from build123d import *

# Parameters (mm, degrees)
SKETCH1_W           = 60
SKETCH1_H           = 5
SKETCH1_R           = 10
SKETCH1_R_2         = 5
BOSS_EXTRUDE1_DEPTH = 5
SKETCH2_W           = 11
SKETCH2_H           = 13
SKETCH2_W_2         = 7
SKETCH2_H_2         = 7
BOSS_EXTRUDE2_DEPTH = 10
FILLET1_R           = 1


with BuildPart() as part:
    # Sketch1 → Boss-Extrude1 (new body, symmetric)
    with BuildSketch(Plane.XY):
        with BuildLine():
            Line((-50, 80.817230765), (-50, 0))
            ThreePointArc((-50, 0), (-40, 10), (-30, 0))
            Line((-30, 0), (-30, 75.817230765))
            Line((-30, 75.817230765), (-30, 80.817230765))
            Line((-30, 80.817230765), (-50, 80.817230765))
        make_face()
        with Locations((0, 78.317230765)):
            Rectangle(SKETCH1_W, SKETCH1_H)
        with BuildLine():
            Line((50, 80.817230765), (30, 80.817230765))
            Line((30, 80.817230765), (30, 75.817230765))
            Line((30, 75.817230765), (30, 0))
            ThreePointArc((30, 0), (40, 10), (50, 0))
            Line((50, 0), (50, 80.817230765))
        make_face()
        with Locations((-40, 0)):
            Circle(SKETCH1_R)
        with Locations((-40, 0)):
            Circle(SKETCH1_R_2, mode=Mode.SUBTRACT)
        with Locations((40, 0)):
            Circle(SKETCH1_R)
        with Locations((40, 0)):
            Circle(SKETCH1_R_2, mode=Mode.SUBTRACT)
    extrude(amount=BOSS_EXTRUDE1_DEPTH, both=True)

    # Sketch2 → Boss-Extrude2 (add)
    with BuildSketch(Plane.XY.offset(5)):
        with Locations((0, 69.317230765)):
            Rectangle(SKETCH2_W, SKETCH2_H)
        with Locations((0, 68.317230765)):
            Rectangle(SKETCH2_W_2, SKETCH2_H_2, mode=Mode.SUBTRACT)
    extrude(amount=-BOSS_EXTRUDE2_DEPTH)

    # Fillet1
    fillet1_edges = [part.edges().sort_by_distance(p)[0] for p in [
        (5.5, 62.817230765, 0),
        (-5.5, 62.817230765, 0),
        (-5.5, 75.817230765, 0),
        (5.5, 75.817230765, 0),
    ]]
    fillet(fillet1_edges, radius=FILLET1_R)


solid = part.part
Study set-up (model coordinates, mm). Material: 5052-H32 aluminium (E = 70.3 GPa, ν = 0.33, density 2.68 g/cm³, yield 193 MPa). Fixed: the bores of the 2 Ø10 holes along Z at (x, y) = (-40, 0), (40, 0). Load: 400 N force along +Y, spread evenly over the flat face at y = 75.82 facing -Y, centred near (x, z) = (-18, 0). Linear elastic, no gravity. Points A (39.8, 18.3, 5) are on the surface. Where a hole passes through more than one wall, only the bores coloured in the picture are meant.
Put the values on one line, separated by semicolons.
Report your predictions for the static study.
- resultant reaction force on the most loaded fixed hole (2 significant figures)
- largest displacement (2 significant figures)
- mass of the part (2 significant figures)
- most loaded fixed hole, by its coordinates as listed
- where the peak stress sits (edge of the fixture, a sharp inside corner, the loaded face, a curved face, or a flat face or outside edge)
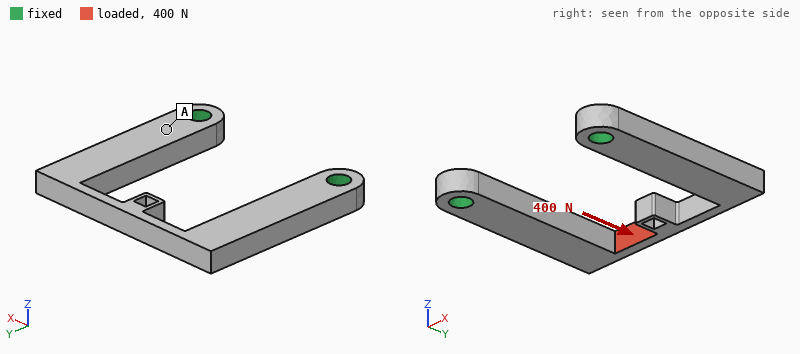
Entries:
340 N; 46 µm; 100 g; (-40, 0); the loaded face
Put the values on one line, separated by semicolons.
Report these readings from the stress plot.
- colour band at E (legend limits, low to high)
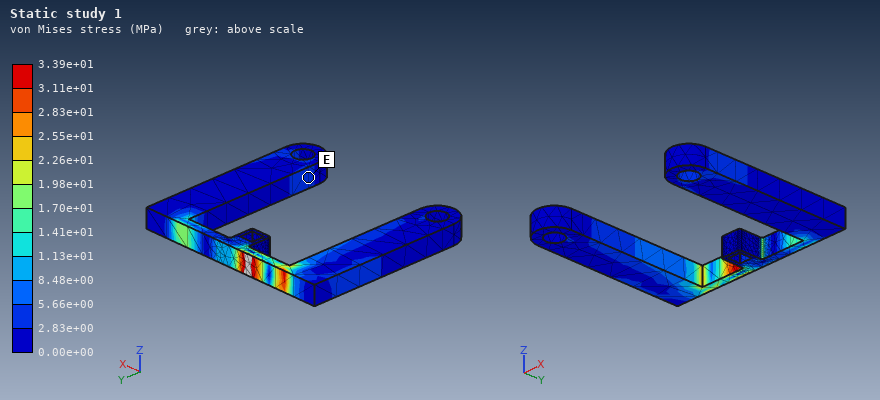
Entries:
2.83e+00 to 5.66e+00 MPa
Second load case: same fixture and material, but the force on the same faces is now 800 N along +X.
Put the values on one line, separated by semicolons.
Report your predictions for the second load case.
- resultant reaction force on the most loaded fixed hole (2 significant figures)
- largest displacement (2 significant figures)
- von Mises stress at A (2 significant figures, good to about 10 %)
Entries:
420 N; 0.17 mm; 5.3 MPa
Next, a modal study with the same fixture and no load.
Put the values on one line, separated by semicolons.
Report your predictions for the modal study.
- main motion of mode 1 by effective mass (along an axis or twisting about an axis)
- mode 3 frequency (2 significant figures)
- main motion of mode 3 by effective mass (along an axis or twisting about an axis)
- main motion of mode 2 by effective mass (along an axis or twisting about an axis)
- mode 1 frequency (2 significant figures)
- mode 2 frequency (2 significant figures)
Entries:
along Z; 2000 Hz; along X; twisting about Y; 1100 Hz; 1800 Hz
